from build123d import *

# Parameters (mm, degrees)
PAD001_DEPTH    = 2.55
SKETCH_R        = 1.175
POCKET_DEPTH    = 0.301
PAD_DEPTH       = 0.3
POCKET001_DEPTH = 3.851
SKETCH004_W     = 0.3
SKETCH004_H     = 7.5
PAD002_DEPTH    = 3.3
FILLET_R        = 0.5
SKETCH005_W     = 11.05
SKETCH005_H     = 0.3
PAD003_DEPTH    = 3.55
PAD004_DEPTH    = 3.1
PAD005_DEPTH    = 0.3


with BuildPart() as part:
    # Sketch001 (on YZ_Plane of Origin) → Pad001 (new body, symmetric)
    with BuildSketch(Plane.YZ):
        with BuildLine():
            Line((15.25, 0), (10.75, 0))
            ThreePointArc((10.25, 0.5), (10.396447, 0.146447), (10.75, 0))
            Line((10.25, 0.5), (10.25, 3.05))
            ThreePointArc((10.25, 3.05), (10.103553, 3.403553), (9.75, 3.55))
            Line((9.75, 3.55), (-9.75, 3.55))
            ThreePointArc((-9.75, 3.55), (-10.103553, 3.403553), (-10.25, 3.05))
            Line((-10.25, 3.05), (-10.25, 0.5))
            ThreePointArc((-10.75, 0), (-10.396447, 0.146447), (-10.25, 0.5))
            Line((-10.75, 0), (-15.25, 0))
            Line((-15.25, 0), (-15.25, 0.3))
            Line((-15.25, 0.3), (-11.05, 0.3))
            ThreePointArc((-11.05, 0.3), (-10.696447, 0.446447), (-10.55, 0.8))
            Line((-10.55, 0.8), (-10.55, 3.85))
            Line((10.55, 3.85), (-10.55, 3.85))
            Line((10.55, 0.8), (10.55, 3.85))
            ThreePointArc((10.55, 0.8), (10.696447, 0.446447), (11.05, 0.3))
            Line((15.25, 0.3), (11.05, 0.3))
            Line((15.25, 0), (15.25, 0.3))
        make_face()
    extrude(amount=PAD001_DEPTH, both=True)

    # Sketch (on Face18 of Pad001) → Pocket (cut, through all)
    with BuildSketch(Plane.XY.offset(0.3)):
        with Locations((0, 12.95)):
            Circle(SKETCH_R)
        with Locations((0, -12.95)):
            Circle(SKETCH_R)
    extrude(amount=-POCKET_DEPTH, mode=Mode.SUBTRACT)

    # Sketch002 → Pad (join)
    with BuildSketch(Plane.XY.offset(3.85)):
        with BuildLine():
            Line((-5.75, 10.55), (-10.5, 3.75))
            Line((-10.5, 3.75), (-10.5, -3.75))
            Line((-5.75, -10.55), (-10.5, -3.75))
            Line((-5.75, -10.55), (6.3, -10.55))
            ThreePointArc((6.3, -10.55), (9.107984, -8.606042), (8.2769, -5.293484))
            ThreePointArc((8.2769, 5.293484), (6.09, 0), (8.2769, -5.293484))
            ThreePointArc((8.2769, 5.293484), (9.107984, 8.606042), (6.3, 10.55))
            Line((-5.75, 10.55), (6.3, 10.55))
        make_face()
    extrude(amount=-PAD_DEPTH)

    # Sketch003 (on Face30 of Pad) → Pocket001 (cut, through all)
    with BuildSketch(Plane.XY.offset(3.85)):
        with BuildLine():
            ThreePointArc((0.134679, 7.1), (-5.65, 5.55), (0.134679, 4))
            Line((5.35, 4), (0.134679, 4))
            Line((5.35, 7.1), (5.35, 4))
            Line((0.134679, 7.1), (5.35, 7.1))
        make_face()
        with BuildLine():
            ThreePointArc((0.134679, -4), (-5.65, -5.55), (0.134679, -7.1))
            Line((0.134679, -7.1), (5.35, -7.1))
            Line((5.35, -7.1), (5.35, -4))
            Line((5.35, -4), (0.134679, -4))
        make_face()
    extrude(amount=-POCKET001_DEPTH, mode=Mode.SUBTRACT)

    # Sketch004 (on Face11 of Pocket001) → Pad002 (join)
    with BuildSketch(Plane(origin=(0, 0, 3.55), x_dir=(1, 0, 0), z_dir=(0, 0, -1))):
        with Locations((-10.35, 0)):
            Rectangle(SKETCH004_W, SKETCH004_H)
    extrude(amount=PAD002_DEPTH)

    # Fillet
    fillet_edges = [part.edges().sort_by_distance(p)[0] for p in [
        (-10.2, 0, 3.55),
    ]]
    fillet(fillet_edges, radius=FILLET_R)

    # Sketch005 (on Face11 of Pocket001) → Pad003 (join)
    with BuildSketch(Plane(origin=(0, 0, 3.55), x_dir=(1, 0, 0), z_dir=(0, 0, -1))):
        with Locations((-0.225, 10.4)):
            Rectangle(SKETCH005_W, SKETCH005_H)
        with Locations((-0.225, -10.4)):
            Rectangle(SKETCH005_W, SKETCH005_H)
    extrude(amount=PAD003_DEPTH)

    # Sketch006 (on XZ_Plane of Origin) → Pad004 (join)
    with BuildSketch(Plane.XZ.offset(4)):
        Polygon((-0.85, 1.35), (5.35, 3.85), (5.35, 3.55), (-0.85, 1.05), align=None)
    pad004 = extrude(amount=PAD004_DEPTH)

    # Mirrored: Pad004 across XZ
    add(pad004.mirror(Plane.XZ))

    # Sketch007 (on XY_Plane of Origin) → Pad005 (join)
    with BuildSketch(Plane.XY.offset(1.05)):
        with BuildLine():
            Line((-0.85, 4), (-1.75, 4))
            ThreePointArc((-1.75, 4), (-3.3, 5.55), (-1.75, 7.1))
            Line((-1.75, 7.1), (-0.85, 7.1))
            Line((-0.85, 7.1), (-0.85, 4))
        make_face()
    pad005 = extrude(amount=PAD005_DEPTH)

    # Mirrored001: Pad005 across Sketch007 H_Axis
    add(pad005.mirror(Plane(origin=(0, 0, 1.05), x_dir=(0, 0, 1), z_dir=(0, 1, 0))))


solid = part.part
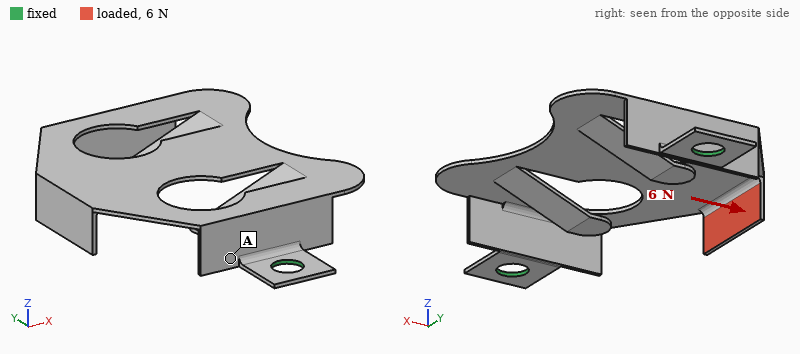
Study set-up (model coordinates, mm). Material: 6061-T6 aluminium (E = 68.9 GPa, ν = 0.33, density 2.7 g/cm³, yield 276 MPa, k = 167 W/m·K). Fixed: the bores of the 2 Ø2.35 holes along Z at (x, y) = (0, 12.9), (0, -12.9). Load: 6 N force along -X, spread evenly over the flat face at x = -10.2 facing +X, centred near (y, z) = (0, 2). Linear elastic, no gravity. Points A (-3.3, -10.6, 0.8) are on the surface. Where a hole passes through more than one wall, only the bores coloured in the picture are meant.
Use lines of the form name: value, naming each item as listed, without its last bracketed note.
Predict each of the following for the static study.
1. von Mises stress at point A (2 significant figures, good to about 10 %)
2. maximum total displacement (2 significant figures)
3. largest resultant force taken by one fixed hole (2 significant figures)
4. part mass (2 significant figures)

von Mises stress at point A: 13 MPa
maximum total displacement: 0.28 mm
largest resultant force taken by one fixed hole: 3.0 N
part mass: 0.37 g
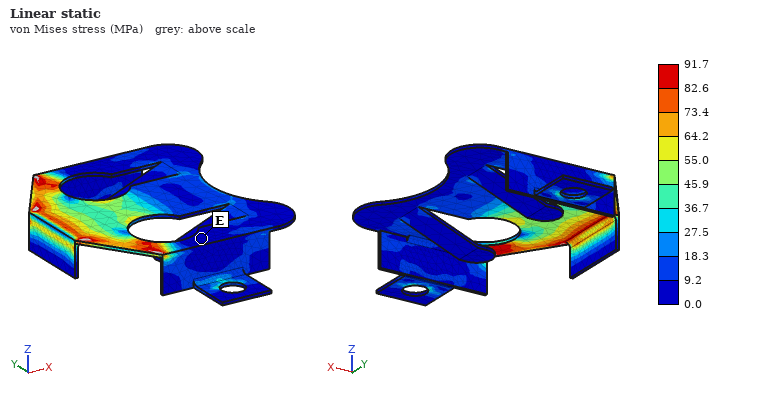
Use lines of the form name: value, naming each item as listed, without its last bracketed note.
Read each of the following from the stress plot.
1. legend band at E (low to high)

legend band at E: 0.0 to 9.2 MPa
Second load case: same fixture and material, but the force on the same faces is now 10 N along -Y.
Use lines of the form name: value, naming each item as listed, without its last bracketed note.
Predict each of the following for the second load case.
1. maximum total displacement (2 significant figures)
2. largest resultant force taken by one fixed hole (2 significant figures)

maximum total displacement: 0.34 mm
largest resultant force taken by one fixed hole: 7.2 N
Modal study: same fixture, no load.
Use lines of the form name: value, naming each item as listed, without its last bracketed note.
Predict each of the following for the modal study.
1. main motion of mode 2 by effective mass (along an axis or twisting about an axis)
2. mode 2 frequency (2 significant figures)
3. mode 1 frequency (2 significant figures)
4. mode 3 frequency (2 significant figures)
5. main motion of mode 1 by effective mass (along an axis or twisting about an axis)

main motion of mode 2 by effective mass: along Z
mode 2 frequency: 2300 Hz
mode 1 frequency: 1800 Hz
mode 3 frequency: 2500 Hz
main motion of mode 1 by effective mass: along Z
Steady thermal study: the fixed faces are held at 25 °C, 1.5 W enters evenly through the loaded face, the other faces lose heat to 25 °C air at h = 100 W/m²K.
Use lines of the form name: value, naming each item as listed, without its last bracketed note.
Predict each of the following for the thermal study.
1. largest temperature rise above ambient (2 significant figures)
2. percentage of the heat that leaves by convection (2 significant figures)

largest temperature rise above ambient: 37 K
percentage of the heat that leaves by convection: 60 %
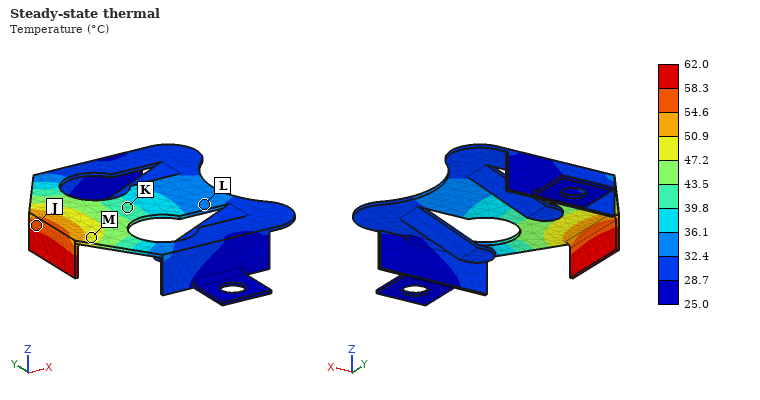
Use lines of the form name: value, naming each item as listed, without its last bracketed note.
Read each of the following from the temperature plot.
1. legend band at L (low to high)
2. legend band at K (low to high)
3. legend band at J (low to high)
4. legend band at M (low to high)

legend band at L: 32.4 to 36.1 °C
legend band at K: 39.8 to 43.5 °C
legend band at J: 54.6 to 58.3 °C
legend band at M: 47.2 to 50.9 °C
